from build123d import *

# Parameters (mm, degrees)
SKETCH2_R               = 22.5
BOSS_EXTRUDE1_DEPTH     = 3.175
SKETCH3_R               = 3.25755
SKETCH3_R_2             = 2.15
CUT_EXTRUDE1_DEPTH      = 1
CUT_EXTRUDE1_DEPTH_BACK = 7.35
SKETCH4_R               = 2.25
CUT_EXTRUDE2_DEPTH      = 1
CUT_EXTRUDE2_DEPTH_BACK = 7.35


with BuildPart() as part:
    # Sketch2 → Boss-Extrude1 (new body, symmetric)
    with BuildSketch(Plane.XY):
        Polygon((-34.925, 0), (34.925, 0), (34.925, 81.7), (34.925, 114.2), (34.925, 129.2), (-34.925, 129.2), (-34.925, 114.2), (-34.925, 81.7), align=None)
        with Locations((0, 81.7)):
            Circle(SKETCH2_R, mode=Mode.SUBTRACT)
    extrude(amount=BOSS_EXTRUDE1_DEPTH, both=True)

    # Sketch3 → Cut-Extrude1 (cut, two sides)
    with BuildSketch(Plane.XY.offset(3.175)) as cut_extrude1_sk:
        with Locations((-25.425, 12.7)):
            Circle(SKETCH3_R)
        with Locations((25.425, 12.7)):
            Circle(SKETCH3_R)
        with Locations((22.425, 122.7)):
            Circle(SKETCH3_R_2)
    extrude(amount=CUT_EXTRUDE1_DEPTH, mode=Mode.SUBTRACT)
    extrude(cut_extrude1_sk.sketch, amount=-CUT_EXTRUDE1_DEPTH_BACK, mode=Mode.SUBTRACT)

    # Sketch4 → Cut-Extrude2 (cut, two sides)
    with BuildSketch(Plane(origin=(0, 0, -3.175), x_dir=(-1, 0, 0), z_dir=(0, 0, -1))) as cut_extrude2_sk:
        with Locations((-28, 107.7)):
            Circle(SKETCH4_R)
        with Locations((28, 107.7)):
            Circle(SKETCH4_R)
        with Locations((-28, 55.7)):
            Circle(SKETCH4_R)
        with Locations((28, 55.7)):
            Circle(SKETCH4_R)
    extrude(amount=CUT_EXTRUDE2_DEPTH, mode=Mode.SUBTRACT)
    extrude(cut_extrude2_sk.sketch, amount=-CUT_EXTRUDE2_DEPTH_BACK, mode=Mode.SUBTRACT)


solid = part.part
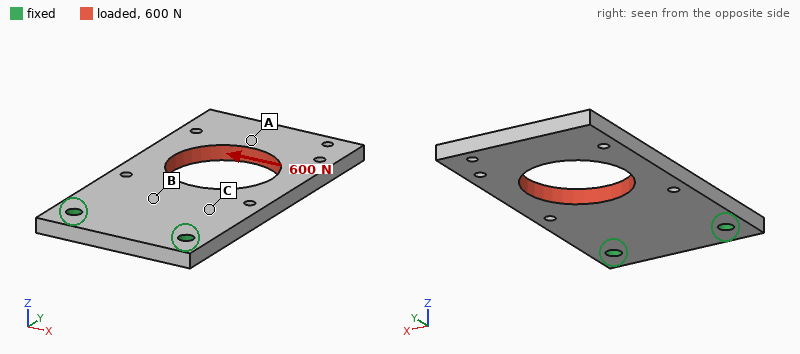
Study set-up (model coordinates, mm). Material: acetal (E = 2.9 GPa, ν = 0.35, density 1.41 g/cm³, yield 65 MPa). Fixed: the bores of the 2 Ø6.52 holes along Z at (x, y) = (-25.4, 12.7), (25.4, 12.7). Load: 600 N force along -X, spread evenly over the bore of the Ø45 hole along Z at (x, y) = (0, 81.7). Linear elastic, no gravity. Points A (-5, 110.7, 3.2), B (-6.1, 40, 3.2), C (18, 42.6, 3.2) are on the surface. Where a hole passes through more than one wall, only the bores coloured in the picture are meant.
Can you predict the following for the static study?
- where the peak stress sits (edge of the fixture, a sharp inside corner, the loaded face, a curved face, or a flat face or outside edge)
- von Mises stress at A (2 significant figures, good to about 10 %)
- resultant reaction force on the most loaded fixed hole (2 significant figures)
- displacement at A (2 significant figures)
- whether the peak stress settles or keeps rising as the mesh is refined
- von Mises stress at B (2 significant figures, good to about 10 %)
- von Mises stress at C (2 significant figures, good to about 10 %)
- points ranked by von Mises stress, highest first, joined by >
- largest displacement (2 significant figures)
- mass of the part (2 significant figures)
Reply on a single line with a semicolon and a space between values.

edge of the fixture; 1.4 MPa; 830 N; 0.61 mm; keeps rising; 4.8 MPa; 2.3 MPa; B > C > A; 0.70 mm; 65 g
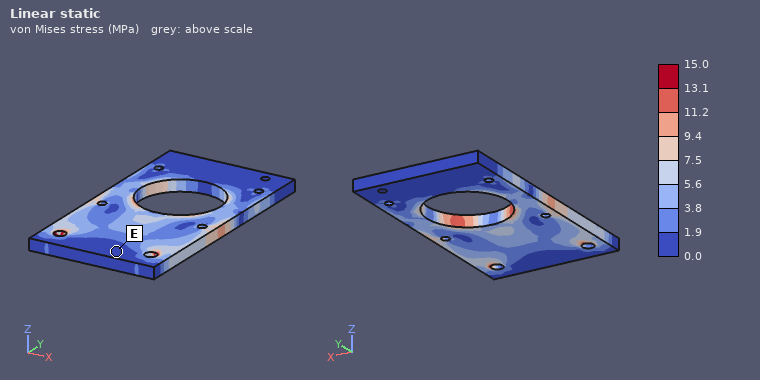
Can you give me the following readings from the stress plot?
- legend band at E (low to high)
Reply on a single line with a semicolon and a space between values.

0.0 to 1.9 MPa
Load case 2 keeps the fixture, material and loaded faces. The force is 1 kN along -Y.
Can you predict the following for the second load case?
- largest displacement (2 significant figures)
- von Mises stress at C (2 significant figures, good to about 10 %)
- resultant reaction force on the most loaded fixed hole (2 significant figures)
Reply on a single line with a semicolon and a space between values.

0.14 mm; 2.3 MPa; 500 N
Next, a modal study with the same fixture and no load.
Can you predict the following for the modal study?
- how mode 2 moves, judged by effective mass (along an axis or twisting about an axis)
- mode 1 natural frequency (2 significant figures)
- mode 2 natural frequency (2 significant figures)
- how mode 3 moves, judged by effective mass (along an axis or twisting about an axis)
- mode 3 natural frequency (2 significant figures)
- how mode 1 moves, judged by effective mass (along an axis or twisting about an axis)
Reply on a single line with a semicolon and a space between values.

twisting about Y; 110 Hz; 340 Hz; along Z; 600 Hz; along Z
